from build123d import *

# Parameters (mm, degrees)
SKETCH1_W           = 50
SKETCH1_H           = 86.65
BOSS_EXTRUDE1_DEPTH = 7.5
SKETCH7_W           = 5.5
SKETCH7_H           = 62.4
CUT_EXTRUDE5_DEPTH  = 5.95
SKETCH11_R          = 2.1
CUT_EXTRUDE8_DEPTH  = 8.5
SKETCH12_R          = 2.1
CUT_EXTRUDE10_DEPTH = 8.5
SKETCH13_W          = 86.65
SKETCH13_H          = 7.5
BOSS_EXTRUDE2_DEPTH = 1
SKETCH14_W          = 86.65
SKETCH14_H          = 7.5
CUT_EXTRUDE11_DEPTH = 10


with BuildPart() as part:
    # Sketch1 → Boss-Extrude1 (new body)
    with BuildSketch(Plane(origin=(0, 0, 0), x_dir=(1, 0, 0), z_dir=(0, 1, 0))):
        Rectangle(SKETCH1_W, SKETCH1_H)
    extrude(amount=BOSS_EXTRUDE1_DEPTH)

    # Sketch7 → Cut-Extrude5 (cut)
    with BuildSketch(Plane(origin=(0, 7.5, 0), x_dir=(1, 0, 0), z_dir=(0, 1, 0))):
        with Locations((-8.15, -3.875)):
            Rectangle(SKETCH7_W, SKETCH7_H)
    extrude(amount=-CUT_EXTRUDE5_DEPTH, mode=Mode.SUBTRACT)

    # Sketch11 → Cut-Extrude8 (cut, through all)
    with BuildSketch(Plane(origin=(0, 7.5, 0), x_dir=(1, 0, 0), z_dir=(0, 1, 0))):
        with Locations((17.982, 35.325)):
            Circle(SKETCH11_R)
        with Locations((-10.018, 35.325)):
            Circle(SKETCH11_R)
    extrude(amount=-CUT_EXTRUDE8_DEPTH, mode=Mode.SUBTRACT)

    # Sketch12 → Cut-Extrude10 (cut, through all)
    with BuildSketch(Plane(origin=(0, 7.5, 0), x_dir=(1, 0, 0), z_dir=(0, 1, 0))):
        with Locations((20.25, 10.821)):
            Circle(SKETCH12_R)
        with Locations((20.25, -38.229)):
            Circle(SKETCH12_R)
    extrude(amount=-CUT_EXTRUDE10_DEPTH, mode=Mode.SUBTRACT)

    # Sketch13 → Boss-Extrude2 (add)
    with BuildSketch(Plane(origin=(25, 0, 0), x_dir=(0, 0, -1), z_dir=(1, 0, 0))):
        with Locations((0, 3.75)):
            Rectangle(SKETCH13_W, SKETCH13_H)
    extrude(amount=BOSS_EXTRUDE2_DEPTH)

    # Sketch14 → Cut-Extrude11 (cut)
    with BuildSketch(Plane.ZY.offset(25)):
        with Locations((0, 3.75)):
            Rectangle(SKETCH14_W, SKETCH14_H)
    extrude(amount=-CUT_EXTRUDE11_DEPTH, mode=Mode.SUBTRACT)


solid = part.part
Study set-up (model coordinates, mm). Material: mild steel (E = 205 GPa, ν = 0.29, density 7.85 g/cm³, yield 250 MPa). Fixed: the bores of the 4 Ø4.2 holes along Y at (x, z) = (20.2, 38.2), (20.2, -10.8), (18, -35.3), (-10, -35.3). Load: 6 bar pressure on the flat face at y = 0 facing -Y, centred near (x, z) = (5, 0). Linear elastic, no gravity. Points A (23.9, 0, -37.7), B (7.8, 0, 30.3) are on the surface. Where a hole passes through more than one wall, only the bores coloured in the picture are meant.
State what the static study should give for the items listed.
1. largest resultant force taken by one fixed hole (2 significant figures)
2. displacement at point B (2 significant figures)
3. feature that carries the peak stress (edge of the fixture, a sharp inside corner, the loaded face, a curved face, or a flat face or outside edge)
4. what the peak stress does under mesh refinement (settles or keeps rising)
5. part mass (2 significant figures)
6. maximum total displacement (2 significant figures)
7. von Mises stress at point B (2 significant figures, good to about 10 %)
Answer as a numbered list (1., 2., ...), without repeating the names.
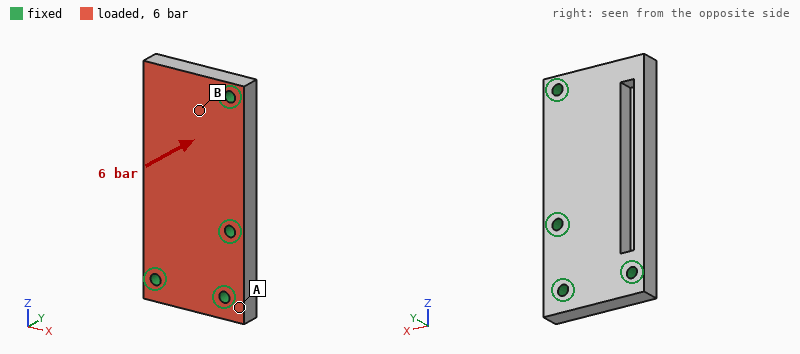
1. 750 N
2. 7.1 µm
3. edge of the fixture
4. keeps rising
5. 190 g
6. 24 µm
7. 15 MPa
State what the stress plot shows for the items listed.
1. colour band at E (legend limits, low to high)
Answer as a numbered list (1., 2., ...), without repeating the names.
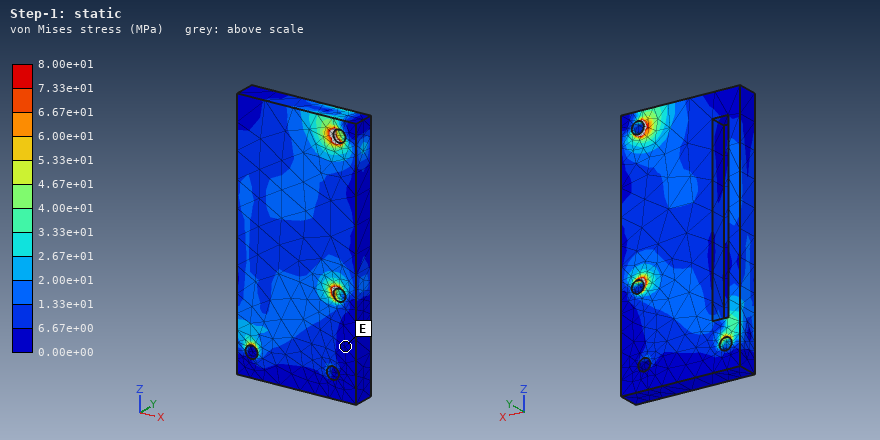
1. 0.00e+00 to 6.67e+00 MPa
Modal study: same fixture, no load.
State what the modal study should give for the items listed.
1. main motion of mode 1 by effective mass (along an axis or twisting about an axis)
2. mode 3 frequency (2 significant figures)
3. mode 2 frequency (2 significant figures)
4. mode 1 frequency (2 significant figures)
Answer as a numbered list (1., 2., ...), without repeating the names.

1. along Y
2. 12 kHz
3. 9900 Hz
4. 4800 Hz
